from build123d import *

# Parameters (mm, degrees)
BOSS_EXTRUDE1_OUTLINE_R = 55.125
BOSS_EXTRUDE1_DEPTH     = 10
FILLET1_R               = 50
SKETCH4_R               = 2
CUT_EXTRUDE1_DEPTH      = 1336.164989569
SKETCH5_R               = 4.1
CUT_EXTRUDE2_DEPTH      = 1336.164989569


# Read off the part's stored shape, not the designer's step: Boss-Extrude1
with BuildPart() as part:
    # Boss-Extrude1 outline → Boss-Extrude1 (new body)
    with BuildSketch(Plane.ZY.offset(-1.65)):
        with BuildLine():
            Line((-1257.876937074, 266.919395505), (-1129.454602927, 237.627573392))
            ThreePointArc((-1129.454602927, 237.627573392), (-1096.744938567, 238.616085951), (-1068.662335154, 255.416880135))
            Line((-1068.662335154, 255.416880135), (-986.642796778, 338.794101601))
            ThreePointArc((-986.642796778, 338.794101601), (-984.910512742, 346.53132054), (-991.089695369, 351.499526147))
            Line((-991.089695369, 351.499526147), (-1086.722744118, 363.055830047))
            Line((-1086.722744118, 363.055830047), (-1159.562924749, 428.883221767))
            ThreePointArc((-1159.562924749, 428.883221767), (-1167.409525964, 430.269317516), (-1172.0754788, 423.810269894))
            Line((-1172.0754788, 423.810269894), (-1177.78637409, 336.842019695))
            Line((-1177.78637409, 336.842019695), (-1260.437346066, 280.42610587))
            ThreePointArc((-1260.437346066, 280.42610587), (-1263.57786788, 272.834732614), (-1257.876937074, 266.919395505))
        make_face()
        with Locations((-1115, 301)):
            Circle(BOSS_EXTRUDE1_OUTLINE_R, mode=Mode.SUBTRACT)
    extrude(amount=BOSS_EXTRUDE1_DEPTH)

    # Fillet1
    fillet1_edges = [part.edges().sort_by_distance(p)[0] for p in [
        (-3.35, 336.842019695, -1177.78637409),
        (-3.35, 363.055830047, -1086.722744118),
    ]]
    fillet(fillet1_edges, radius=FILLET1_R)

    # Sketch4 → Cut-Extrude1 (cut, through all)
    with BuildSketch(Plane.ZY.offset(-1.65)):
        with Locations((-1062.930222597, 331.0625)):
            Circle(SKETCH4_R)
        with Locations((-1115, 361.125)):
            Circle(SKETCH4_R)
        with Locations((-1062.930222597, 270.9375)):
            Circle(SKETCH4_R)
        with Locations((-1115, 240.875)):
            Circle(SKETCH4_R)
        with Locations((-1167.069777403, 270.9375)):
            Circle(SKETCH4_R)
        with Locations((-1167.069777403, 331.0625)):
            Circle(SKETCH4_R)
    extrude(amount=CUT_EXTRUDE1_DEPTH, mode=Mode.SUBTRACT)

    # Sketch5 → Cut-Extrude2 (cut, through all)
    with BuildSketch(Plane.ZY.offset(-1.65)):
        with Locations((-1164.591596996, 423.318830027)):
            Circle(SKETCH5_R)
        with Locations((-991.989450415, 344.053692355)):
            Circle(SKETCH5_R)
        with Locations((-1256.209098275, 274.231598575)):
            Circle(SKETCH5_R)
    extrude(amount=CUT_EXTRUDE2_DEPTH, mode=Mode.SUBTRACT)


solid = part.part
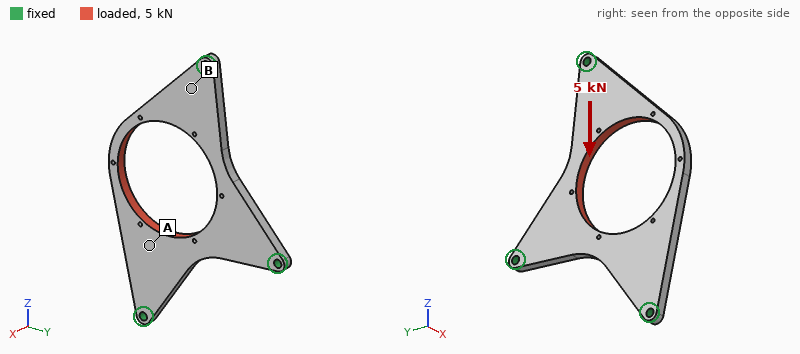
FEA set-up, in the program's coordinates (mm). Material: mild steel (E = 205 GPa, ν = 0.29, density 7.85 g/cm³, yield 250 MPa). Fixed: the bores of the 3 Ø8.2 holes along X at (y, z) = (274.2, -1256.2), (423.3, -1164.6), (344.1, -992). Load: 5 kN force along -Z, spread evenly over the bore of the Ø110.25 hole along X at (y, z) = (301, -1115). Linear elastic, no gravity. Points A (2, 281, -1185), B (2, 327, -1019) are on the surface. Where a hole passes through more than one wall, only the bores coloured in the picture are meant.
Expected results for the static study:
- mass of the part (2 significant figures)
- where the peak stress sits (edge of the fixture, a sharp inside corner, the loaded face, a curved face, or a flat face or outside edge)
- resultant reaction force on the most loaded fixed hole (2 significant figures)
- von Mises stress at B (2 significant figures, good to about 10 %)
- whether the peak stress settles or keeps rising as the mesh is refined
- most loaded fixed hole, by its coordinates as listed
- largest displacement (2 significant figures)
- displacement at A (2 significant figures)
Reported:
1.2 kg
edge of the fixture
2.6 kN
3.9 MPa
keeps rising
(274.2, -1256.2)
14 µm
2.3 µm
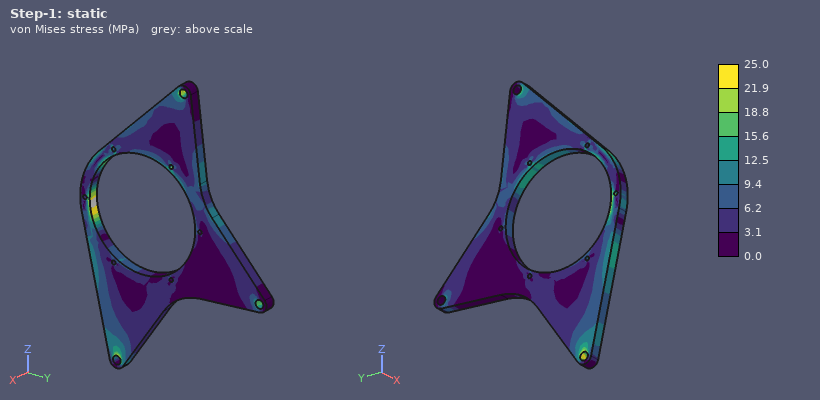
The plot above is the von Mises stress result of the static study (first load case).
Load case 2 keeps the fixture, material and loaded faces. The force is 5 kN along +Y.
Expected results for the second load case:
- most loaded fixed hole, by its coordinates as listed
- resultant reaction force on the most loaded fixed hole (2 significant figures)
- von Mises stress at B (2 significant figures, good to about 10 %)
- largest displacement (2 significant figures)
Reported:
(423.3, -1164.6)
3.4 kN
6.2 MPa
12 µm
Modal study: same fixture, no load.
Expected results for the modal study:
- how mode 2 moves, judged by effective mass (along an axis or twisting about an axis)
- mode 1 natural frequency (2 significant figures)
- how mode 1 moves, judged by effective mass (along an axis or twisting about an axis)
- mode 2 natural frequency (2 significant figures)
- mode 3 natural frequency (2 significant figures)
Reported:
along X
630 Hz
along X
1300 Hz
1400 Hz
